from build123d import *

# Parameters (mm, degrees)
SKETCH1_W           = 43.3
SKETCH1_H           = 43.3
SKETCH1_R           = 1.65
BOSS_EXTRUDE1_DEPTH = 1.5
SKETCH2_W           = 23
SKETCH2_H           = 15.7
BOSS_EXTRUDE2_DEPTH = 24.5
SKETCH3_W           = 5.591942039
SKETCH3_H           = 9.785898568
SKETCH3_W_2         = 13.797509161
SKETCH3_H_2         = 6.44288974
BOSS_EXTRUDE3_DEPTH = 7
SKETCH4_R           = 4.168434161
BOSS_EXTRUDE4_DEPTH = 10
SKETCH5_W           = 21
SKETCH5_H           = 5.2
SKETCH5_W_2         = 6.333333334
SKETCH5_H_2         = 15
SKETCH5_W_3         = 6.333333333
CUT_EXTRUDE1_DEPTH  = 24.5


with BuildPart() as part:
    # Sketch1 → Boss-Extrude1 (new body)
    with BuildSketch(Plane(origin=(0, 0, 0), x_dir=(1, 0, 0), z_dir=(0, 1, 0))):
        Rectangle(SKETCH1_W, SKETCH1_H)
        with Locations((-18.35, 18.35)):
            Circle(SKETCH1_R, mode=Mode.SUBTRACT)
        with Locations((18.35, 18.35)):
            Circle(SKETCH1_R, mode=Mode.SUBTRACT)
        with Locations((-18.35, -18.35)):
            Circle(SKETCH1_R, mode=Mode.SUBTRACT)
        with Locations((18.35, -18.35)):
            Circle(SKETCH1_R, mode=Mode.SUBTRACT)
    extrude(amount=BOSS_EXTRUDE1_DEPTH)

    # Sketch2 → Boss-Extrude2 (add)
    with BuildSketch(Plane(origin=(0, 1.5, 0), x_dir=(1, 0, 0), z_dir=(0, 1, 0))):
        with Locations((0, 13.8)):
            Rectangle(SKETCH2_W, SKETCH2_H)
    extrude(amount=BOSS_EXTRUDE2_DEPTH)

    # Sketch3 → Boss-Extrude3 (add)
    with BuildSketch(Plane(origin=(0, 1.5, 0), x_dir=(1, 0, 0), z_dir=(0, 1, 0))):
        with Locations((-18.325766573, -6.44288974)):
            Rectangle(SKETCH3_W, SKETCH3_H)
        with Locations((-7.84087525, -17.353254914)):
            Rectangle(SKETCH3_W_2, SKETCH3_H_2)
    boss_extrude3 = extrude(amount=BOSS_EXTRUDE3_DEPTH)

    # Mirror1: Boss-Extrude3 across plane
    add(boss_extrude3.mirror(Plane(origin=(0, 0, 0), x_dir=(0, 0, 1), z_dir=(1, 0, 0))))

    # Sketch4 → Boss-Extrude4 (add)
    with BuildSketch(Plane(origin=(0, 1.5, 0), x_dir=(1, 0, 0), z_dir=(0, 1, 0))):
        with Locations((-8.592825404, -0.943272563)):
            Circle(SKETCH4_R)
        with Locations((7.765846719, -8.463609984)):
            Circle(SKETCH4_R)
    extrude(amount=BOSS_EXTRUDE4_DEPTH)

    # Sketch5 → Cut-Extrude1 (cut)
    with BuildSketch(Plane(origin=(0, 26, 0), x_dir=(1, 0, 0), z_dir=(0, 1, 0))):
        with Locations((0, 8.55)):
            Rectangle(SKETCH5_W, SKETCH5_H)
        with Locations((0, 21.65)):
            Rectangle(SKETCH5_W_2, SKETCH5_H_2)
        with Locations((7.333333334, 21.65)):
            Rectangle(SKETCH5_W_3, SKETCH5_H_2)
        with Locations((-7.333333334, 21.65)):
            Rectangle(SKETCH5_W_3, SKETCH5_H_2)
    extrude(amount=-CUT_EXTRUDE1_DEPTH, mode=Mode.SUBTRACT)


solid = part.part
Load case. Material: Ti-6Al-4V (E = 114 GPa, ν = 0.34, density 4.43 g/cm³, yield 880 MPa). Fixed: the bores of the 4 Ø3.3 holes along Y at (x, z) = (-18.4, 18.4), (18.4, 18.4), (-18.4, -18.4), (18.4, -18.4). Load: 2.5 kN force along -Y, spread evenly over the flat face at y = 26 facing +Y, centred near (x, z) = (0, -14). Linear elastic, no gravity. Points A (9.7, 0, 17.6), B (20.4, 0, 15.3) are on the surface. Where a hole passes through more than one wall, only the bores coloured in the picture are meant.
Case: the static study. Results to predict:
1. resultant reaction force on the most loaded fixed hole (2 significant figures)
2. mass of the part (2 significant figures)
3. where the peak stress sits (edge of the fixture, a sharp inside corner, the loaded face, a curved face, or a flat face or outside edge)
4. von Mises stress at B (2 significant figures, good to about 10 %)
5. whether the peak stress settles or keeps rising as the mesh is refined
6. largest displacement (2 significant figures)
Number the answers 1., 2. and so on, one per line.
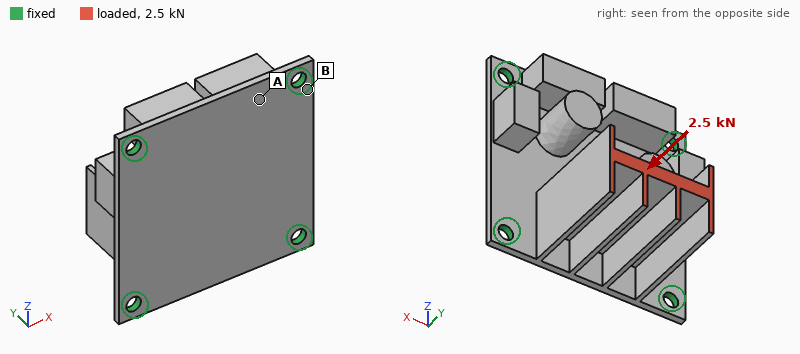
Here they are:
1. 1.2 kN
2. 38 g
3. edge of the fixture
4. 150 MPa
5. keeps rising
6. 0.27 mm
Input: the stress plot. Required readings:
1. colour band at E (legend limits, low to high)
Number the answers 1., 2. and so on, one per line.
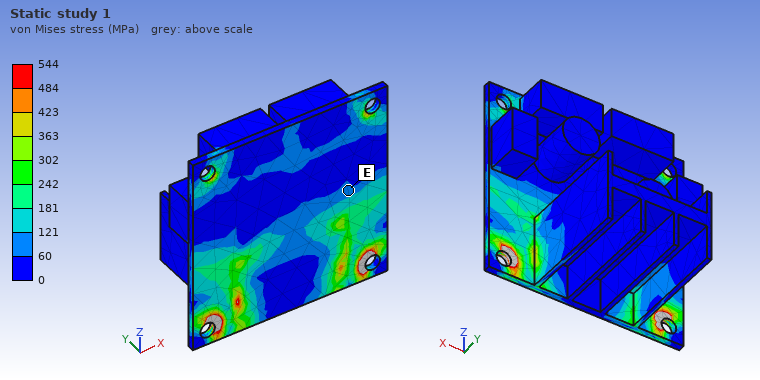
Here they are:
1. 60 to 121 MPa
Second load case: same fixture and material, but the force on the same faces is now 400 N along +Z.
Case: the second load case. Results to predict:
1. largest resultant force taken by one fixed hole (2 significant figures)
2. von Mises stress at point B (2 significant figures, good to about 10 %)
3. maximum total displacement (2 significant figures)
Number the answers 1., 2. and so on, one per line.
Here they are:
1. 180 N
2. 130 MPa
3. 0.40 mm
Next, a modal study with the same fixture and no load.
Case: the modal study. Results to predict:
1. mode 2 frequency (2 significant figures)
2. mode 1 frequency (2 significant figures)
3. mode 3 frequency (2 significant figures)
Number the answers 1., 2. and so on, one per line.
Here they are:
1. 4400 Hz
2. 2200 Hz
3. 4400 Hz
